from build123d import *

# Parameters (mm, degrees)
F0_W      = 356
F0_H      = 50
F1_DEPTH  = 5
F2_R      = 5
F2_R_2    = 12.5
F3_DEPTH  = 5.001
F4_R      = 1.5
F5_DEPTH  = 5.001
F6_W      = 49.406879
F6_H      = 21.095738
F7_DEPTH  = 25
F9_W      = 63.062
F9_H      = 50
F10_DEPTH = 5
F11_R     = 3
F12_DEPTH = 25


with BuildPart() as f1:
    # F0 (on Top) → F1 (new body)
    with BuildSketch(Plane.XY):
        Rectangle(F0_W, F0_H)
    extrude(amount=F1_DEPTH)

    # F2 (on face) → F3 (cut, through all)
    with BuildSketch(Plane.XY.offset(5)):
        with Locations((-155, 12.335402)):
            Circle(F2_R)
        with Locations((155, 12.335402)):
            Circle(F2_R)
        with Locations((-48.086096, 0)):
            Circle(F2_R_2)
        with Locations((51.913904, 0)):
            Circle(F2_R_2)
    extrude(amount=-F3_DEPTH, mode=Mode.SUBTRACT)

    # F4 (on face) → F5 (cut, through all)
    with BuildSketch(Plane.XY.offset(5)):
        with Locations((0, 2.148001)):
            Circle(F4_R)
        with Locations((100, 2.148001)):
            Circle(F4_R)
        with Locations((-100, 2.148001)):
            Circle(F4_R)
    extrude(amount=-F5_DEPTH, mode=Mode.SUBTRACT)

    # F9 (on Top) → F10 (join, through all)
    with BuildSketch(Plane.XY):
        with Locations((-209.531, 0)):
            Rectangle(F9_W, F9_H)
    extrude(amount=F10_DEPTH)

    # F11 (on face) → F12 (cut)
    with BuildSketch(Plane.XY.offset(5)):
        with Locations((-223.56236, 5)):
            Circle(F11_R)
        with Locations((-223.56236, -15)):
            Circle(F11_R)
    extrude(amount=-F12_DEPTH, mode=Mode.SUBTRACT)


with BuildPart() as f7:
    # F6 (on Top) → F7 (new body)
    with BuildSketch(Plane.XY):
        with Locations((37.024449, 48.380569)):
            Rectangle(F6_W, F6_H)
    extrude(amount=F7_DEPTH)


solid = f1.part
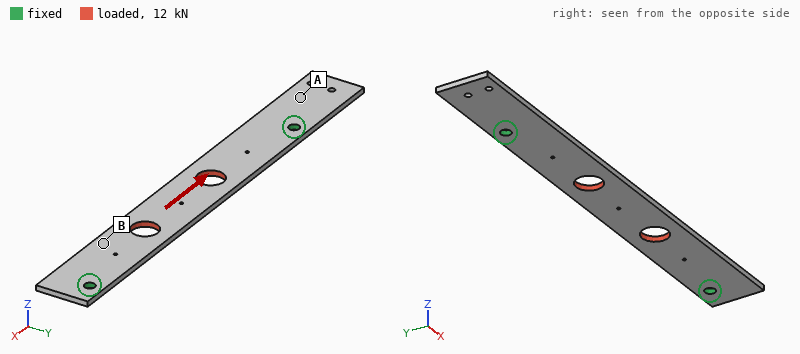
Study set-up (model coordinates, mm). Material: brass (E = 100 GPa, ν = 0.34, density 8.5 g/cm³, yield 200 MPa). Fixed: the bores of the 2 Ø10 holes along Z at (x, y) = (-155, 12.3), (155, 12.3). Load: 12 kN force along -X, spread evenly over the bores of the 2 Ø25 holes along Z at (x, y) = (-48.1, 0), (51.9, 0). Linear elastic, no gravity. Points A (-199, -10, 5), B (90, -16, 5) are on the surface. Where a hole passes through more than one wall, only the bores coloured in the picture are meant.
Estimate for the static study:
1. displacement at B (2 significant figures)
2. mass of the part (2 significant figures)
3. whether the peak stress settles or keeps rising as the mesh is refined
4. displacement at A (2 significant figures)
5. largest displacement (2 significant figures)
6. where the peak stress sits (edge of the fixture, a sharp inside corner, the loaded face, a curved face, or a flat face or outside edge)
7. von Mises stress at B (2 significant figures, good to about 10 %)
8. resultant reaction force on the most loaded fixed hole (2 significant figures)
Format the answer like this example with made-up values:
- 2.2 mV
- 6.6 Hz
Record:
- 31 µm
- 840 g
- keeps rising
- 26 µm
- 50 µm
- edge of the fixture
- 17 MPa
- 6.0 kN
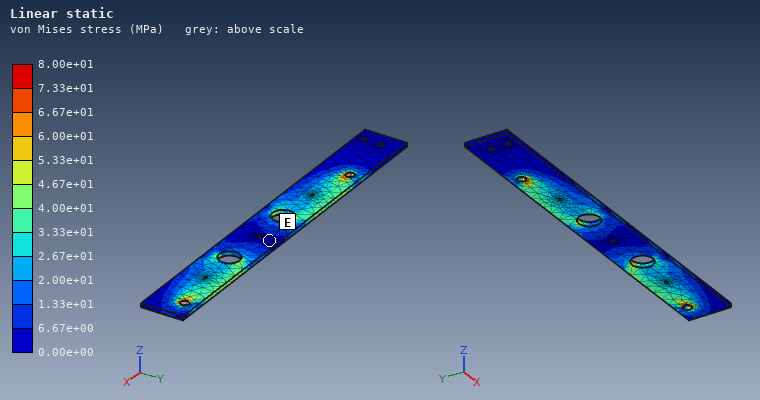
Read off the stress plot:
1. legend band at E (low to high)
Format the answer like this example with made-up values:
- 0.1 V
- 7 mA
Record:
- 0.00e+00 to 6.67e+00 MPa
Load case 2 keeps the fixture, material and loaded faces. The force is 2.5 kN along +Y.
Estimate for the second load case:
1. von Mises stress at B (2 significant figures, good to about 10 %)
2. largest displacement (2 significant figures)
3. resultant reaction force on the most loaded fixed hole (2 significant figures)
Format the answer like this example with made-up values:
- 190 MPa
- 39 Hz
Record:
- 15 MPa
- 0.14 mm
- 1.8 kN
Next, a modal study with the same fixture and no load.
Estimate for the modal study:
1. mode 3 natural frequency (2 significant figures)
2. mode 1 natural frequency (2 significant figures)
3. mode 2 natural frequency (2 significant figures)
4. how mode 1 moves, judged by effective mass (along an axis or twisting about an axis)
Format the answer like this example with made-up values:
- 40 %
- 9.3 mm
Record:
- 490 Hz
- 190 Hz
- 380 Hz
- along Z
